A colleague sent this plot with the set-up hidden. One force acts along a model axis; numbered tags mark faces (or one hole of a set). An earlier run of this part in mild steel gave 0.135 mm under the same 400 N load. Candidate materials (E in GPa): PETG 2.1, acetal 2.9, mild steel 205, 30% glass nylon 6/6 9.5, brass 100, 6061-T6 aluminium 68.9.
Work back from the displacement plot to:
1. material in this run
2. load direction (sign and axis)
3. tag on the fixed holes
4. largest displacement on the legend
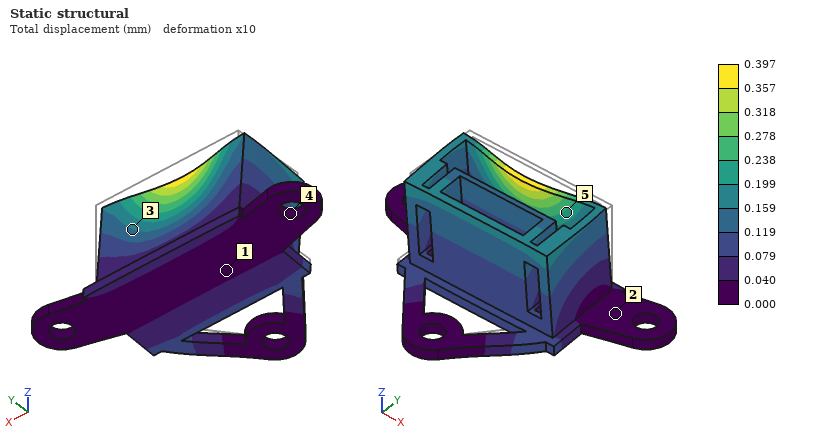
6061-T6 aluminium
-Y
4
0.397 mm
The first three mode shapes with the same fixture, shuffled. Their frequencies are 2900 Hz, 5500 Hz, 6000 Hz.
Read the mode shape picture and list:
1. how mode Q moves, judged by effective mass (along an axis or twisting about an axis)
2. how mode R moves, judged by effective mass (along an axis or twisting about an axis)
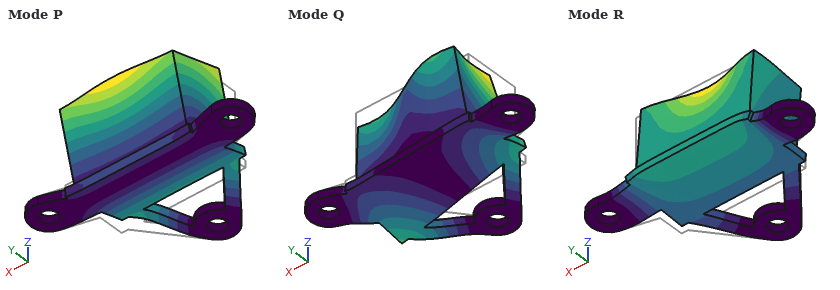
along X
along Z
